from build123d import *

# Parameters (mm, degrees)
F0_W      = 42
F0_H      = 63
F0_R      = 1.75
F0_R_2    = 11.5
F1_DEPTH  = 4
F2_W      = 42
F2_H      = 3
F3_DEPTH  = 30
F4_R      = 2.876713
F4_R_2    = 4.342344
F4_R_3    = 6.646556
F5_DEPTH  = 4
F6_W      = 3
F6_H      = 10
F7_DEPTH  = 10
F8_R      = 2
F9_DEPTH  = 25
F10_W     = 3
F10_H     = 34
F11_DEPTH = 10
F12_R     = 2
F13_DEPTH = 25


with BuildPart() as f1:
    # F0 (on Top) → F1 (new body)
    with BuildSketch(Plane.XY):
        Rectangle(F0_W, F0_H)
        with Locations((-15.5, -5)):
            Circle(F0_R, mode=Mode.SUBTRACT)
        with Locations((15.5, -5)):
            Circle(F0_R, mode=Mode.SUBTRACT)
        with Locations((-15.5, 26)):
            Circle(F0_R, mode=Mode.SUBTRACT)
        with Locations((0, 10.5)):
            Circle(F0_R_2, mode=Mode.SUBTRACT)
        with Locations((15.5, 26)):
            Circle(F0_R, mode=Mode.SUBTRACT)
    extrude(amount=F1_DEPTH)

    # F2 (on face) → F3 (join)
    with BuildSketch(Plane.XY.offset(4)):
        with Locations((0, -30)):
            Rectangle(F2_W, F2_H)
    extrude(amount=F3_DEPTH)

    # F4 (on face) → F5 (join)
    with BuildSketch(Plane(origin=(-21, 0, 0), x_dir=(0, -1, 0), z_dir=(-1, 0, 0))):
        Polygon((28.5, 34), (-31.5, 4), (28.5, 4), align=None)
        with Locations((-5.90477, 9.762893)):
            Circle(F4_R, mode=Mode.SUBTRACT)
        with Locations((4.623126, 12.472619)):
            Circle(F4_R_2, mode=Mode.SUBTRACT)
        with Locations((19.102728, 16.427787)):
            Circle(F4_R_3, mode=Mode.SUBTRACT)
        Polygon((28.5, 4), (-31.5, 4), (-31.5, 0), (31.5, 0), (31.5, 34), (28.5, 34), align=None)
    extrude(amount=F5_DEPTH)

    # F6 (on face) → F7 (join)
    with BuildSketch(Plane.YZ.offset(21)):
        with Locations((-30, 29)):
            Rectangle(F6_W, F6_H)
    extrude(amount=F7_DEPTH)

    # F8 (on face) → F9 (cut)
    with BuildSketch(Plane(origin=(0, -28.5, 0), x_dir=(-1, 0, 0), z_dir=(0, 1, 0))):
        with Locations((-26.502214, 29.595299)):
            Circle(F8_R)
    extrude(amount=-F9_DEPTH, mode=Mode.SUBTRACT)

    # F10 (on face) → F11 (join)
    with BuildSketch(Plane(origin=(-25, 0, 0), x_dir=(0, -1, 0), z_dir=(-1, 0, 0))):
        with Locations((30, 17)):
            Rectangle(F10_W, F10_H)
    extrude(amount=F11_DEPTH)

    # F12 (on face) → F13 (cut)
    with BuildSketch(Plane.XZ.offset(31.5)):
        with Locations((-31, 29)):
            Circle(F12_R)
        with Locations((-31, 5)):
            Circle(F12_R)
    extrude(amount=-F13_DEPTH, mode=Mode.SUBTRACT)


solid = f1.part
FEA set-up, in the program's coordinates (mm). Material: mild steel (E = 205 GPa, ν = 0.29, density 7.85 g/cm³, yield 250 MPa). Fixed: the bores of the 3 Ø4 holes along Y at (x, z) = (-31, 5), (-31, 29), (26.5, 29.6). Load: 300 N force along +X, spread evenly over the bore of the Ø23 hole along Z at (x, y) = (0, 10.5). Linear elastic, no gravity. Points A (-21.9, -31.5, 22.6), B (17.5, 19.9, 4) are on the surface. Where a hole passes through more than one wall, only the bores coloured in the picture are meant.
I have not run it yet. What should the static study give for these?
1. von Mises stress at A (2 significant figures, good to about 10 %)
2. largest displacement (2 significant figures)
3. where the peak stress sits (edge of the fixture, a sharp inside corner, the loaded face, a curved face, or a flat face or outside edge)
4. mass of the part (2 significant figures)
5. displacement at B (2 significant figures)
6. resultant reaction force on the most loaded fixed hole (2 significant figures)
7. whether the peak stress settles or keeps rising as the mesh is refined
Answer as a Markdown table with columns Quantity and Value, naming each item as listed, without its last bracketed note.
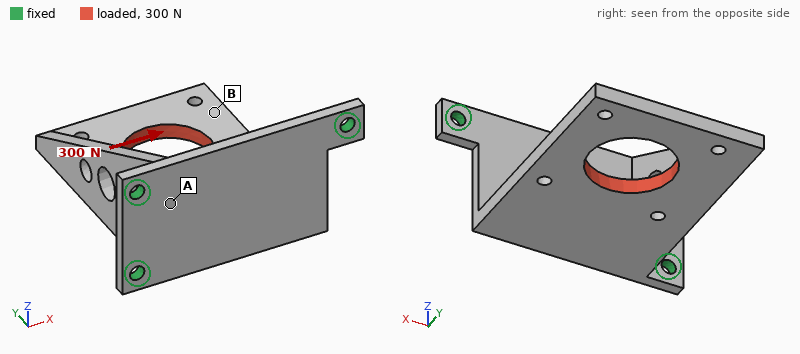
| Quantity | Value |
|---|---|
| von Mises stress at A | 19 MPa |
| largest displacement | 0.16 mm |
| where the peak stress sits | edge of the fixture |
| mass of the part | 140 g |
| displacement at B | 0.13 mm |
| resultant reaction force on the most loaded fixed hole | 230 N |
| whether the peak stress settles or keeps rising as the mesh is refined | keeps rising |
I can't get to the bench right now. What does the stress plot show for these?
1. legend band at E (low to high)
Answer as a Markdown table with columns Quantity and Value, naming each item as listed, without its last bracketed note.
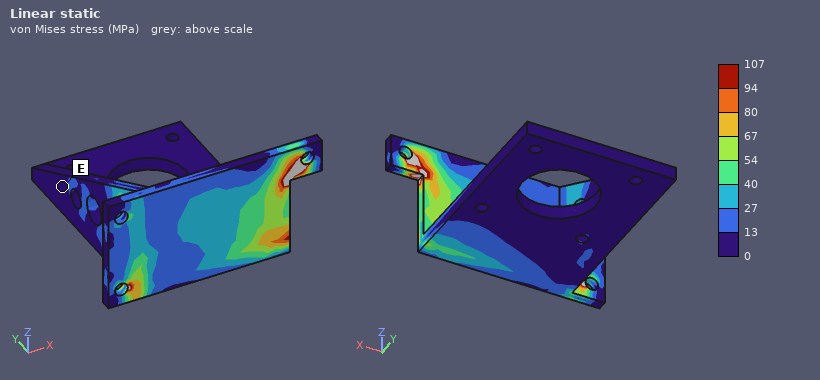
| Quantity | Value |
|---|---|
| legend band at E | 0 to 13 MPa |
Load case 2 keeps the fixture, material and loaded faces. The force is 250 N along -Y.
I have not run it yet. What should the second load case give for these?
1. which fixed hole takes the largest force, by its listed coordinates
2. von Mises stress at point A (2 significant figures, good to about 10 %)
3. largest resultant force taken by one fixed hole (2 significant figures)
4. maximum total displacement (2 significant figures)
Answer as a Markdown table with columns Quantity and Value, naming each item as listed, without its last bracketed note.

| Quantity | Value |
|---|---|
| which fixed hole takes the largest force, by its listed coordinates | (-31, 5) |
| von Mises stress at point A | 13 MPa |
| largest resultant force taken by one fixed hole | 230 N |
| maximum total displacement | 88 µm |
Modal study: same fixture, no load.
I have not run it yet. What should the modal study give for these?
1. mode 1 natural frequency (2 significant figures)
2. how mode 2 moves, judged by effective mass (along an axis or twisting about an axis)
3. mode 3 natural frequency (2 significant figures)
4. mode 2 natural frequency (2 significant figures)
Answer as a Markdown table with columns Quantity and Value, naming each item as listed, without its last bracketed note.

| Quantity | Value |
|---|---|
| mode 1 natural frequency | 930 Hz |
| how mode 2 moves, judged by effective mass | along Z |
| mode 3 natural frequency | 3400 Hz |
| mode 2 natural frequency | 1500 Hz |
